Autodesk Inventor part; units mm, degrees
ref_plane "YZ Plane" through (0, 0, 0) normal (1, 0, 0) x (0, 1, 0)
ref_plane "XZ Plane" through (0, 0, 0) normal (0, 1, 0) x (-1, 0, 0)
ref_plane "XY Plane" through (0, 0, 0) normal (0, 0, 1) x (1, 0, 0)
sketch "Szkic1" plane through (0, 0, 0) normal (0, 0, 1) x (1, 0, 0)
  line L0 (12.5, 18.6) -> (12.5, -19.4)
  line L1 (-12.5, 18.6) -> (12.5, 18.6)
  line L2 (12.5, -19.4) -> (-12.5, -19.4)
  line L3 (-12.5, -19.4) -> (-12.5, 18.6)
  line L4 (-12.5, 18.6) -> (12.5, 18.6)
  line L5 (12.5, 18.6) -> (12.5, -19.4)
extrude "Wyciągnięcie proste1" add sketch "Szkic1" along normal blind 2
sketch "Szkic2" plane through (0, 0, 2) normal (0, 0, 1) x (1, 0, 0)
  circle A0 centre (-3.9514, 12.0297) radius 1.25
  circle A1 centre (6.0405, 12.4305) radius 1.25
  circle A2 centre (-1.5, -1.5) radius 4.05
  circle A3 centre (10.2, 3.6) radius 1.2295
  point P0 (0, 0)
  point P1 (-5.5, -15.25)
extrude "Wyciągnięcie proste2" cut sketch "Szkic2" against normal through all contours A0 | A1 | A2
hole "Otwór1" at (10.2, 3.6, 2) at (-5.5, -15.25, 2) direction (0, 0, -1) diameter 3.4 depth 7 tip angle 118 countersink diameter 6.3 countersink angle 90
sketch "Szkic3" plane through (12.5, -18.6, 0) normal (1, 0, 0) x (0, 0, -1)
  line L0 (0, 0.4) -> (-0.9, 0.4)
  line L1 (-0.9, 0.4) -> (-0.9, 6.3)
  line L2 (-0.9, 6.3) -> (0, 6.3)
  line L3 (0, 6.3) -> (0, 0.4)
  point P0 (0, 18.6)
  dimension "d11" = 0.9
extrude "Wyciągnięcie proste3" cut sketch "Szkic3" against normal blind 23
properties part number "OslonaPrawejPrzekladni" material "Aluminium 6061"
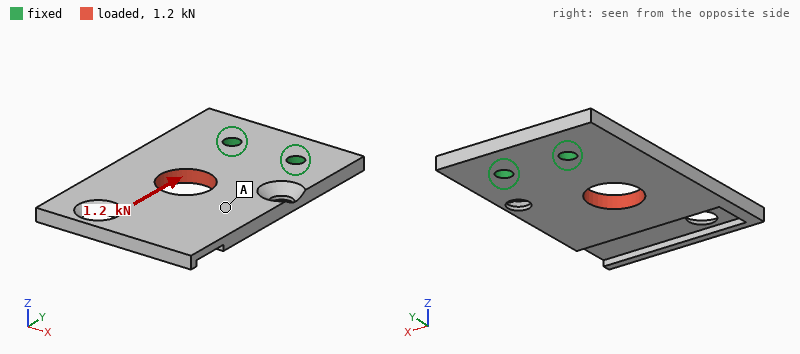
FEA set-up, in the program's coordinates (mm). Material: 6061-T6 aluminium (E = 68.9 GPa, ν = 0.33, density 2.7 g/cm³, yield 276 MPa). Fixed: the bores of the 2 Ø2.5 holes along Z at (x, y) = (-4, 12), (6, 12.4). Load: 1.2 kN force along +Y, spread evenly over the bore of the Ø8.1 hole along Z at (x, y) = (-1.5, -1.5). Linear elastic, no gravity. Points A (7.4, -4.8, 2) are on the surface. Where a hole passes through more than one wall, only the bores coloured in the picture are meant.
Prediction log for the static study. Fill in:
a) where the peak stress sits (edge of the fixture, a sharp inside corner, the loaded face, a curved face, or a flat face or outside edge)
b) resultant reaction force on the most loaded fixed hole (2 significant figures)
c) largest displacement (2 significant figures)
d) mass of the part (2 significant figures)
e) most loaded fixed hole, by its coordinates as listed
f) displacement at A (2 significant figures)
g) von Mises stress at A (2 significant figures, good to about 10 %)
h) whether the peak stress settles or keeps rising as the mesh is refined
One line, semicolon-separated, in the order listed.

edge of the fixture; 860 N; 16 µm; 4.3 g; (-4, 12); 6.4 µm; 10.0 MPa; keeps rising
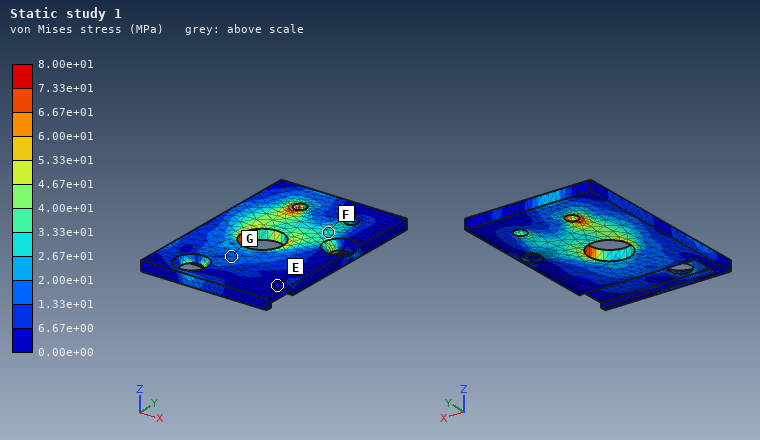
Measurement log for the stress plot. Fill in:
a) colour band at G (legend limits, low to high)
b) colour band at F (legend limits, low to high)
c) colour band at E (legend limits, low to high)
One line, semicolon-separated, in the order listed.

1.33e+01 to 2.00e+01 MPa; 2.67e+01 to 3.33e+01 MPa; 0.00e+00 to 6.67e+00 MPa
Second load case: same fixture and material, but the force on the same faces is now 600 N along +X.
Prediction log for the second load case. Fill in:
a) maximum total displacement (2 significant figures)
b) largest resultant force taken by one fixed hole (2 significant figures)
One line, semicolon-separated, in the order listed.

44 µm; 760 N
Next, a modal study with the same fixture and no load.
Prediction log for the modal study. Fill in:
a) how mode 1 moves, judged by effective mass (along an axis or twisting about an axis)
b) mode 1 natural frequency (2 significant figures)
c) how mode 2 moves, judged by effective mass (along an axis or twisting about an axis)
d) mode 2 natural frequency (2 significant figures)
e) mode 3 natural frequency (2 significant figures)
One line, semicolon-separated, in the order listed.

along Z; 1700 Hz; twisting about Y; 4200 Hz; 9500 Hz
